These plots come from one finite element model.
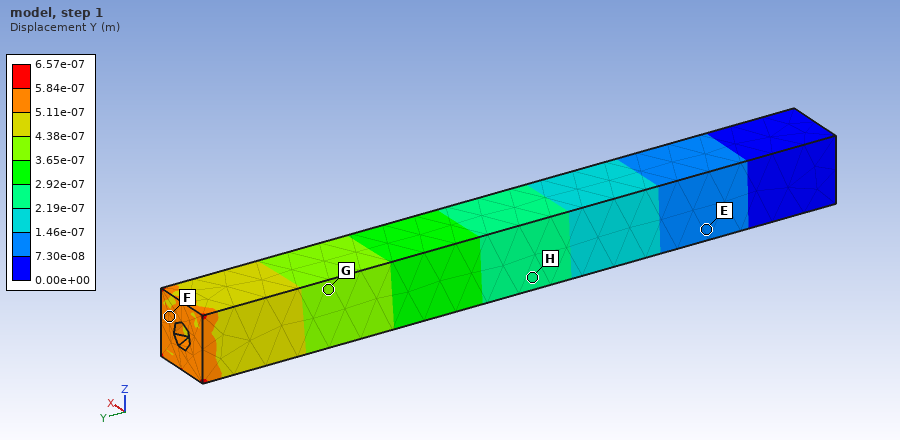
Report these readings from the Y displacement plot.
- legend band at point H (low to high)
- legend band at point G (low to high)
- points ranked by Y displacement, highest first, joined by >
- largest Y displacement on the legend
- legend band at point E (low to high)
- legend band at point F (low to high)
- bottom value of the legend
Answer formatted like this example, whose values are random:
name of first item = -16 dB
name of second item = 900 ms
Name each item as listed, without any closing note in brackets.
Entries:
legend band at point H = 2.19e-07 to 2.92e-07 m
legend band at point G = 3.65e-07 to 4.38e-07 m
points ranked by Y displacement, highest first, joined by > = F > G > H > E
largest Y displacement on the legend = 6.57e-07 m
legend band at point E = 7.30e-08 to 1.46e-07 m
legend band at point F = 5.11e-07 to 5.84e-07 m
bottom value of the legend = 0.00e+00 m
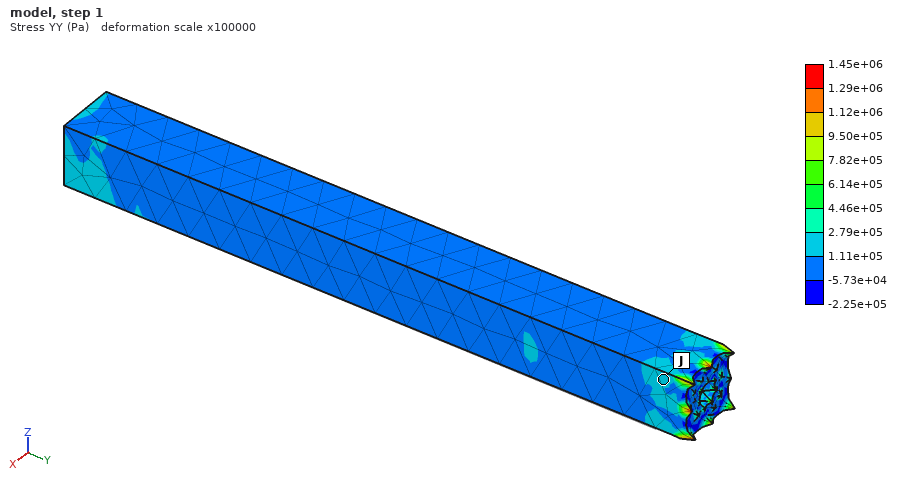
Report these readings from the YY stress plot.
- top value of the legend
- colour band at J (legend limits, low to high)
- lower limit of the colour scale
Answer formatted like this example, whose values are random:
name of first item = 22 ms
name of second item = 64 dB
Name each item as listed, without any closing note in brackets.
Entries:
top value of the legend = 1.45e+06 Pa
colour band at J = 1.11e+05 to 2.79e+05 Pa
lower limit of the colour scale = -2.25e+05 Pa
